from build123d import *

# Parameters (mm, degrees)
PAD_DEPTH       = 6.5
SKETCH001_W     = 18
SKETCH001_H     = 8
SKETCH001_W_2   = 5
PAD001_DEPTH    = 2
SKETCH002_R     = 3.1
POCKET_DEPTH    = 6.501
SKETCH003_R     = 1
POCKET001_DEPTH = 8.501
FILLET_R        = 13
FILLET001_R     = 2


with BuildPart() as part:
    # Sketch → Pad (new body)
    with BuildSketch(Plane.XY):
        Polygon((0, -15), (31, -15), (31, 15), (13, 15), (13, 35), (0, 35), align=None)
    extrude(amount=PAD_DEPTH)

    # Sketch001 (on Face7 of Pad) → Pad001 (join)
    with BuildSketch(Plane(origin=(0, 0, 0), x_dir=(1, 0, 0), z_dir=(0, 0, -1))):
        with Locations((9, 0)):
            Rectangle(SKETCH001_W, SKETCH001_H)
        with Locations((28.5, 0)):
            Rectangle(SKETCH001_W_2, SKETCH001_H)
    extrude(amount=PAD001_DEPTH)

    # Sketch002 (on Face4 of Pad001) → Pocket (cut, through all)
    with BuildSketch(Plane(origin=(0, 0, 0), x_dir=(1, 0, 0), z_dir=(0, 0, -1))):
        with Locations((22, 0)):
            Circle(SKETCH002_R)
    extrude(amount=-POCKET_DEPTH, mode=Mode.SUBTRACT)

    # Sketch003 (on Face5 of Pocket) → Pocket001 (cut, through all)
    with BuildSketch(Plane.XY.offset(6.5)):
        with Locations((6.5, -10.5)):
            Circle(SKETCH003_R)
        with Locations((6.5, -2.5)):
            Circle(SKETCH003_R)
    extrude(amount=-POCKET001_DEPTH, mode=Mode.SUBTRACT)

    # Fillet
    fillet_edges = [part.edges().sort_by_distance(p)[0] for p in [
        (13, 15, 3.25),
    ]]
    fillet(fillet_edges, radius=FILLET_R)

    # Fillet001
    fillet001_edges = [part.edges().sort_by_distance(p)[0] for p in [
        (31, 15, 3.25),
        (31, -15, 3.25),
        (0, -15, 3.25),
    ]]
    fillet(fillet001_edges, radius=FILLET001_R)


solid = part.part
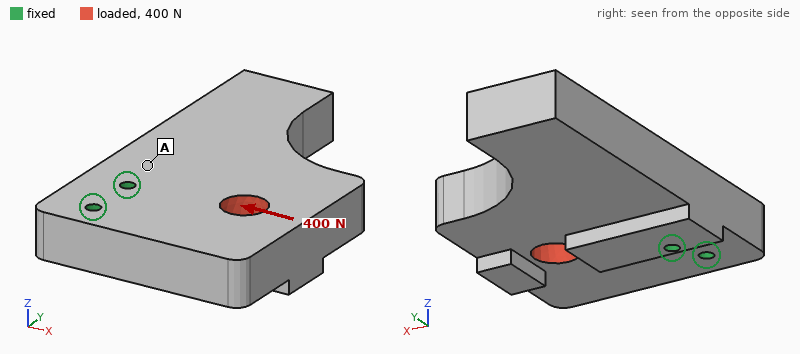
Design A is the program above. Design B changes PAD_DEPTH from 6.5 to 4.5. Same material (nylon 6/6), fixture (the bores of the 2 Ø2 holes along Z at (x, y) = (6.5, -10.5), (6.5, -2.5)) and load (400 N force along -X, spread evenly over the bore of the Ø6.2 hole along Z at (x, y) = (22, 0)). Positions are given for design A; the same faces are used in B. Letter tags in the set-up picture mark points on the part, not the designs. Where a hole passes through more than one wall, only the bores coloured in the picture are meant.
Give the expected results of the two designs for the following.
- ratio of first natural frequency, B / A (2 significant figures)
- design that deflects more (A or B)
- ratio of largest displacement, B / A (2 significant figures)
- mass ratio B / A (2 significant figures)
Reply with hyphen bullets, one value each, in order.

- 0.76
- B
- 1.4
- 0.71
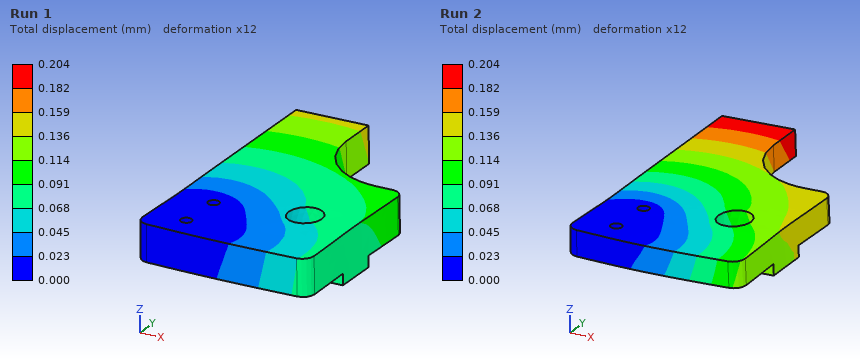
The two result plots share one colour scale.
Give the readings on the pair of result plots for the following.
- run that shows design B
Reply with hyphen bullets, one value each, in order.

- Run 2
